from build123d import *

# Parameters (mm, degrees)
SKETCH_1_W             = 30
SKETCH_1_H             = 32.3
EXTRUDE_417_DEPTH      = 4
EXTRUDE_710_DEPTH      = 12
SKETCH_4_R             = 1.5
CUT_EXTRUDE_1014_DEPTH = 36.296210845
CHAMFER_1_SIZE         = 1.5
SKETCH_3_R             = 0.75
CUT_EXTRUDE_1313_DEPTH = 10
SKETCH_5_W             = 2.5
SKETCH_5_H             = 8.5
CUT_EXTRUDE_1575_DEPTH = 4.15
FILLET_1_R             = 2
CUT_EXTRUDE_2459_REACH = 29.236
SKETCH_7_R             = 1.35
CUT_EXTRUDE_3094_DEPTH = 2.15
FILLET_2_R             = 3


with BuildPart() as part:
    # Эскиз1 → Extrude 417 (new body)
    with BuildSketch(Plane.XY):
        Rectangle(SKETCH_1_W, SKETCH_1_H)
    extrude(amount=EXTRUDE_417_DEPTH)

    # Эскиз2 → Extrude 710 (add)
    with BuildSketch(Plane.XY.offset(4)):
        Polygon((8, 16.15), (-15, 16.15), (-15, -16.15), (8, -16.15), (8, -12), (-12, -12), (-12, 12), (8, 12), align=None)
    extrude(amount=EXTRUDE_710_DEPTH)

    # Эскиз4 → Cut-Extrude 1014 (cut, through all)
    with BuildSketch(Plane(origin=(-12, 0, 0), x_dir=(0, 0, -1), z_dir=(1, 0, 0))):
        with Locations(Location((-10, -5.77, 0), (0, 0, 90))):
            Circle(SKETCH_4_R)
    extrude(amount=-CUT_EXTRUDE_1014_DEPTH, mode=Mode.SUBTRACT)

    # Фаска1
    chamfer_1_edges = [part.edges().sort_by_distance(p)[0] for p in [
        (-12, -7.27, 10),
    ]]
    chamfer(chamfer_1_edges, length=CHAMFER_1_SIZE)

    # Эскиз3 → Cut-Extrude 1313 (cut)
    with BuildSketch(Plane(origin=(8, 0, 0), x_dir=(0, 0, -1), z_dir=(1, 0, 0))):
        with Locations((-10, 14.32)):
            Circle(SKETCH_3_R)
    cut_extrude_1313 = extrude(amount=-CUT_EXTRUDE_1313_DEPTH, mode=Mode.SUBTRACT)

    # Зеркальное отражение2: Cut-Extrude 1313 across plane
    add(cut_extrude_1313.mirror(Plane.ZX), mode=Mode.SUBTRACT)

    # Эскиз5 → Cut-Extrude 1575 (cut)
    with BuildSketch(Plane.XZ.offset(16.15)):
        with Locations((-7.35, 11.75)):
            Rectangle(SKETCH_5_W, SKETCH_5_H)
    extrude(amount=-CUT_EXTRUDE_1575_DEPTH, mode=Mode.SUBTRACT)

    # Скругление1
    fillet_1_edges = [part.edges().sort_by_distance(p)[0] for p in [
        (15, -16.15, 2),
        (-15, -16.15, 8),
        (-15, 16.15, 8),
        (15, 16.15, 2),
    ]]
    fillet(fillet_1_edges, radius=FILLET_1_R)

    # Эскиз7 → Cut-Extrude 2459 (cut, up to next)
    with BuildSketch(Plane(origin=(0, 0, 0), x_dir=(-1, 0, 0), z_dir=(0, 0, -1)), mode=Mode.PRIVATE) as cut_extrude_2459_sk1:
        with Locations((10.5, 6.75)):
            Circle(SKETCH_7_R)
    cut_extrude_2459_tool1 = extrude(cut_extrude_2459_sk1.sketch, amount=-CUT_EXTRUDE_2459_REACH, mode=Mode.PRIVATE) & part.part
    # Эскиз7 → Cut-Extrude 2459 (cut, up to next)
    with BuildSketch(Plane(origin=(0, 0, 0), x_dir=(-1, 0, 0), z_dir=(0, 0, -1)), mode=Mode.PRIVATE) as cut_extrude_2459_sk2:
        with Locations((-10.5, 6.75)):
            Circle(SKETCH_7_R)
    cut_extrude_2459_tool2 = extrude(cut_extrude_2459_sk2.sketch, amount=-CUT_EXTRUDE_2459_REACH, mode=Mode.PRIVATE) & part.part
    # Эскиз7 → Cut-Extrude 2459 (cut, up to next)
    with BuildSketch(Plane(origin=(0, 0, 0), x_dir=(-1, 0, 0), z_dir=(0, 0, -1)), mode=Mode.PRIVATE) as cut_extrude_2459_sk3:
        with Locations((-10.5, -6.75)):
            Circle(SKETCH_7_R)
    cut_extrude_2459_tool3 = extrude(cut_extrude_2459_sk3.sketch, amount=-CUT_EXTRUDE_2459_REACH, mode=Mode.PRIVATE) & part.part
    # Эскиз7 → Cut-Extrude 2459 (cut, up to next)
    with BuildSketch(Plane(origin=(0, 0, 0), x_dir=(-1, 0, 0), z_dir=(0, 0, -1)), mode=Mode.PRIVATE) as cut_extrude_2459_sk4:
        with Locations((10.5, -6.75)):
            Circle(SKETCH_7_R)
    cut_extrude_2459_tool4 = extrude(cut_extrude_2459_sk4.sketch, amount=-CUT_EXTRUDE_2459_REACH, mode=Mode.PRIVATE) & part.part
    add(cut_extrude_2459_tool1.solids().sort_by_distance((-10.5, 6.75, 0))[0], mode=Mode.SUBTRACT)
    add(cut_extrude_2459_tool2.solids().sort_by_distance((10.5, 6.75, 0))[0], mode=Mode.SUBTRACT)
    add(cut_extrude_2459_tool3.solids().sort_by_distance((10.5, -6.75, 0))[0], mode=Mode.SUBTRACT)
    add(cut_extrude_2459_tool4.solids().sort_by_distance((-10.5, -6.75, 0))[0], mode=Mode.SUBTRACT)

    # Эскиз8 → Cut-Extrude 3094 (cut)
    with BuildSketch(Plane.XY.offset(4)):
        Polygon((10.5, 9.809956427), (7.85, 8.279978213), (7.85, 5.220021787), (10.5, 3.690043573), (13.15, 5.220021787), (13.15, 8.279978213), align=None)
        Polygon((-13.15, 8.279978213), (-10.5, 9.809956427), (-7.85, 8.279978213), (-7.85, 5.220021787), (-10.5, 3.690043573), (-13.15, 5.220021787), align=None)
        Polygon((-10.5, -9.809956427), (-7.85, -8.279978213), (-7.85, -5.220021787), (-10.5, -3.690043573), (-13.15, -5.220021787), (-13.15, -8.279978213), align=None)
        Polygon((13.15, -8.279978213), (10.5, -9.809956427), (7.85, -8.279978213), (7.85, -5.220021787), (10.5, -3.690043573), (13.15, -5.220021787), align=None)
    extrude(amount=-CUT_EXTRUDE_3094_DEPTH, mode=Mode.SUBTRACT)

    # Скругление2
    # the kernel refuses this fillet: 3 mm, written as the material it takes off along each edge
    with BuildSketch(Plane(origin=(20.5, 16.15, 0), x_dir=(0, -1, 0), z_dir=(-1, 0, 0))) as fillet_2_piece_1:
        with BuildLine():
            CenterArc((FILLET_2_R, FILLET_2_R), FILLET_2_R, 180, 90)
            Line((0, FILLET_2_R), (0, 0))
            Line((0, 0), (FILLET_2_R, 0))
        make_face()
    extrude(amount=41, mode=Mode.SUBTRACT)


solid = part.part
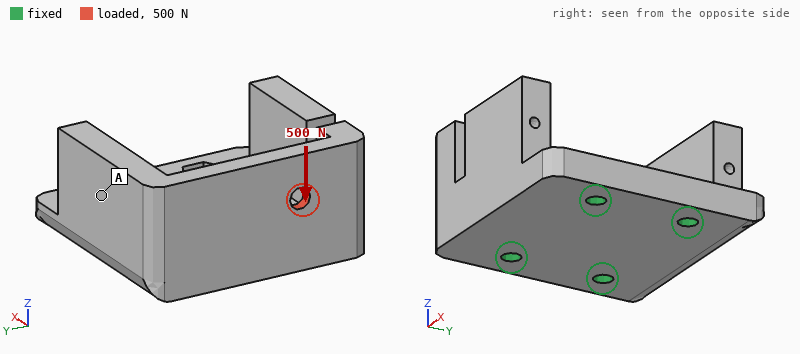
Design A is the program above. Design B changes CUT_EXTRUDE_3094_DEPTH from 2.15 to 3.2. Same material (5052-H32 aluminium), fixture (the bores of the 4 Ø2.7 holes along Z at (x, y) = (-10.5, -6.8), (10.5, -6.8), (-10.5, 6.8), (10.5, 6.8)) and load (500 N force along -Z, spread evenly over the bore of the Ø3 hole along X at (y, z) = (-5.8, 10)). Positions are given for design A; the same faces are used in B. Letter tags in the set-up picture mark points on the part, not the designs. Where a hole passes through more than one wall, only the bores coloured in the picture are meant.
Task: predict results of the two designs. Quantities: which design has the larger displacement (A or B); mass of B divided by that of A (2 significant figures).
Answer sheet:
B
0.99
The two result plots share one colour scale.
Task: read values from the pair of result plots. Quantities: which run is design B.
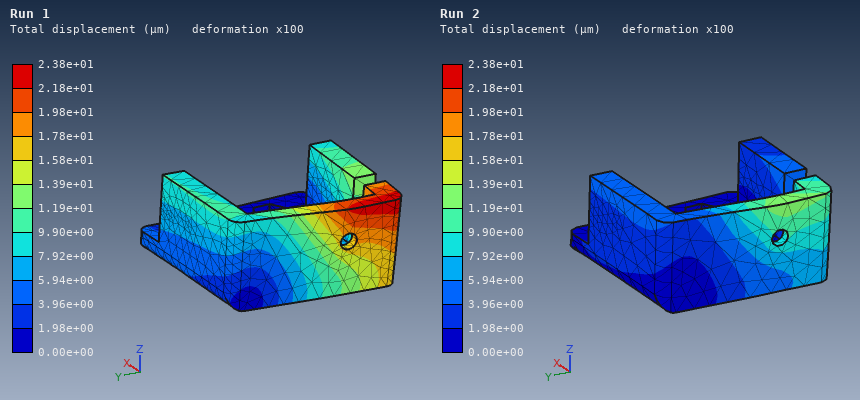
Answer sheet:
Run 1
